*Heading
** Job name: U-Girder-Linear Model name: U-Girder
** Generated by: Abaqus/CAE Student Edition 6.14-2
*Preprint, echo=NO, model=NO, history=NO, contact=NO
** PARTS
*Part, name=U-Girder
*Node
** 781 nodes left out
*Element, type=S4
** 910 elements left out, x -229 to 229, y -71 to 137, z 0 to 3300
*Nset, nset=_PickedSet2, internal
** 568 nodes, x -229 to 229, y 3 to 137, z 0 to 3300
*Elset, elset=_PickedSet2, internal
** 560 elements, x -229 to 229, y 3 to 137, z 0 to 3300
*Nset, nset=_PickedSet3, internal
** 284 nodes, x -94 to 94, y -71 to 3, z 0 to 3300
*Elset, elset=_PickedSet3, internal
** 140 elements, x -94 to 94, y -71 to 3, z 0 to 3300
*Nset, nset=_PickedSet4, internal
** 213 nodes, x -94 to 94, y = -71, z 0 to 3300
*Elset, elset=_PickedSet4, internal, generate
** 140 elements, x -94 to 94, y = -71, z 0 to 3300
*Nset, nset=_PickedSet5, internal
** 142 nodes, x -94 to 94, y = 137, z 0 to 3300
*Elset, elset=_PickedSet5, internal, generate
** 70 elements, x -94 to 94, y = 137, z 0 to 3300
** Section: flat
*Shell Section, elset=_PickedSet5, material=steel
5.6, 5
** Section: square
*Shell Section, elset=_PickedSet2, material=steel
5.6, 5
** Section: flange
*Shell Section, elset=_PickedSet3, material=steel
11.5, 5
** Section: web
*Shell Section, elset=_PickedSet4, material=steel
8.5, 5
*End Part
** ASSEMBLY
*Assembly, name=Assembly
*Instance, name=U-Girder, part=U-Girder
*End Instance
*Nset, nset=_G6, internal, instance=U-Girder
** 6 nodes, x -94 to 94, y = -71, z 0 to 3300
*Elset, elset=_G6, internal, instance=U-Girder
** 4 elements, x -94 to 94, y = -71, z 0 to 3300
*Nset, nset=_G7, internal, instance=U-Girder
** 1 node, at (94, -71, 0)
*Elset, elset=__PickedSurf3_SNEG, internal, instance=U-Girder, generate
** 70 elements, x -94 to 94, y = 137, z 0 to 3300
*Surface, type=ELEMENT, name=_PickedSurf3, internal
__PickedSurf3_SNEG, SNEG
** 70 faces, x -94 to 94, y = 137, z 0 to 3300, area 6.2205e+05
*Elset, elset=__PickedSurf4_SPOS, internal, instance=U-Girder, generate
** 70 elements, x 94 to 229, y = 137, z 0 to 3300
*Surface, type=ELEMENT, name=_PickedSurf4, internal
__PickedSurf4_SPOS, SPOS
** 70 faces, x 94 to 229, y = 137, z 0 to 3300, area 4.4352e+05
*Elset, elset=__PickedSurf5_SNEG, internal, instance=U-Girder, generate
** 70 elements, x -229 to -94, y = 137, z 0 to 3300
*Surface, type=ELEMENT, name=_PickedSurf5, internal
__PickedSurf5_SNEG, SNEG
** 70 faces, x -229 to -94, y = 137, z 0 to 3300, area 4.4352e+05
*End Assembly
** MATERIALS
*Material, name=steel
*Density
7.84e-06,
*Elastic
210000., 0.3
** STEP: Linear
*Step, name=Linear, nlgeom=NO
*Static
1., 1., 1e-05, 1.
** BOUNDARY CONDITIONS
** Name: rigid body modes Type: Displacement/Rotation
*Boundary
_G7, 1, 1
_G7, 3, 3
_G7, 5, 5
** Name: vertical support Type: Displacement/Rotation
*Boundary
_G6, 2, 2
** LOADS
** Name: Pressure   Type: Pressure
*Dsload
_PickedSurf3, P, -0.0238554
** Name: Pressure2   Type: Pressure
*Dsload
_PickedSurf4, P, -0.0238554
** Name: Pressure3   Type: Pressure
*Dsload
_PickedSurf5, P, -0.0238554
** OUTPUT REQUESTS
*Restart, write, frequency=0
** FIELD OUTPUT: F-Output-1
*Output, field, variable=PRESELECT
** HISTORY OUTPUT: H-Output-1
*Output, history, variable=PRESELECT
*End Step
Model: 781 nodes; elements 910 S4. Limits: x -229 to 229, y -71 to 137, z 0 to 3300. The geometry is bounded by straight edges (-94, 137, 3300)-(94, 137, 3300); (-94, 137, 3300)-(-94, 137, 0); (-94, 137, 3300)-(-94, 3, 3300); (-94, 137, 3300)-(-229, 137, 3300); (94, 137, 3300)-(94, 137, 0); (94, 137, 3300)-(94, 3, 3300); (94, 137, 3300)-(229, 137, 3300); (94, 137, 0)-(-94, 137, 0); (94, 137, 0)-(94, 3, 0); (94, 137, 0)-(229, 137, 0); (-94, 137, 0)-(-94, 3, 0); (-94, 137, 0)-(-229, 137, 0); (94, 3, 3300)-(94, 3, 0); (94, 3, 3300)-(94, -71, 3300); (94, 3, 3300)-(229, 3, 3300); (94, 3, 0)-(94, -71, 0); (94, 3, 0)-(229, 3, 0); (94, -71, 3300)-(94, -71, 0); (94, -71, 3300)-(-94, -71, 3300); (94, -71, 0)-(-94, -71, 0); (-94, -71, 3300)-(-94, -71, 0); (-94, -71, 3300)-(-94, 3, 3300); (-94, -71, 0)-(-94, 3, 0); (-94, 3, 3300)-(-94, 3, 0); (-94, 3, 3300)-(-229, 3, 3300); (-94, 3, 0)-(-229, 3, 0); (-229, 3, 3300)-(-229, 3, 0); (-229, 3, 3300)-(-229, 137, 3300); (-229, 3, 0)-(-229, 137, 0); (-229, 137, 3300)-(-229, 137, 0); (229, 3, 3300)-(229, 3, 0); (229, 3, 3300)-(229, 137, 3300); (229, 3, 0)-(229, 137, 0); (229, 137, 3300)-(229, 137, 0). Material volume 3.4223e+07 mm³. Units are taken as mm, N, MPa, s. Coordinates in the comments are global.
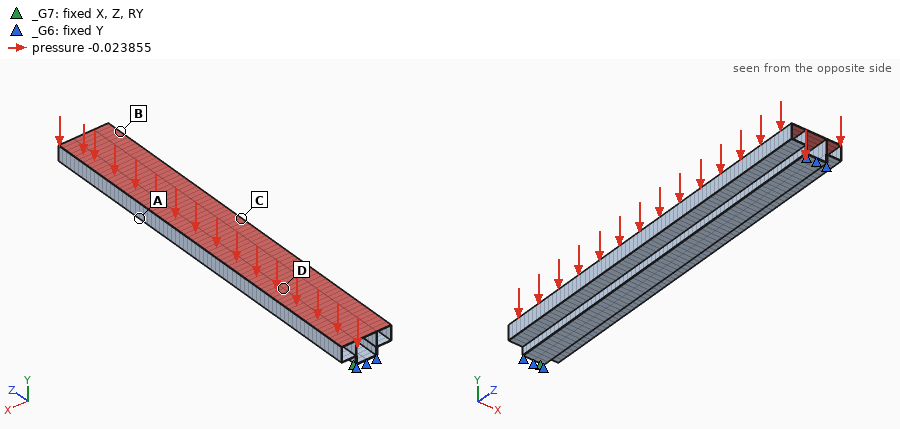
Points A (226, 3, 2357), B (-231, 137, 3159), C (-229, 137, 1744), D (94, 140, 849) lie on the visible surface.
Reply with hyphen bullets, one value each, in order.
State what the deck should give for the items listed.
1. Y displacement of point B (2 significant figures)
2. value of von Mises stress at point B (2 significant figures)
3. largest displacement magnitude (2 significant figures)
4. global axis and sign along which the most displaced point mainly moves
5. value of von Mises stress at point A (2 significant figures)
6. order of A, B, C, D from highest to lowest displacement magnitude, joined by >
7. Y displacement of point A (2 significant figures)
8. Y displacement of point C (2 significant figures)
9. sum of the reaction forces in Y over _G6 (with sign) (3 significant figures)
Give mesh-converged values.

- -0.32 mm
- 6.1 MPa
- 1.5 mm
- -Y
- 8.6 MPa
- C > A > D > B
- -1.1 mm
- -1.4 mm
- 36000 N
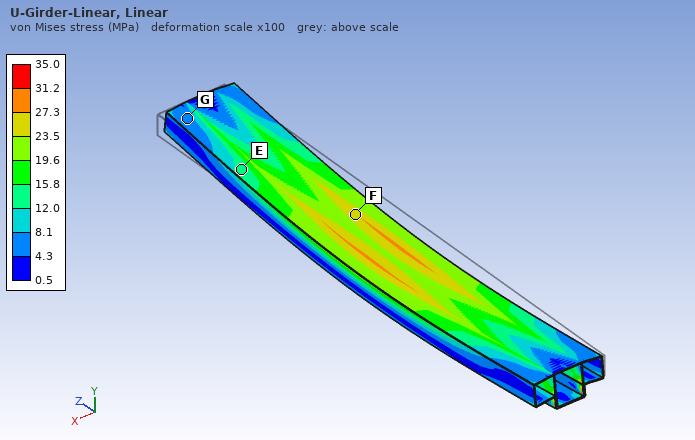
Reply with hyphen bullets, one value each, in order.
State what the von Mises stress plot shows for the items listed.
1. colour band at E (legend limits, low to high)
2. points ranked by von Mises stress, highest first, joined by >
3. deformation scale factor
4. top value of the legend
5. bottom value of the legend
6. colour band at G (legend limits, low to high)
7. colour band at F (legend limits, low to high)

- 12.0 to 15.8 MPa
- F > E > G
- 100
- 35.0 MPa
- 0.5 MPa
- 4.3 to 8.1 MPa
- 23.5 to 27.3 MPa
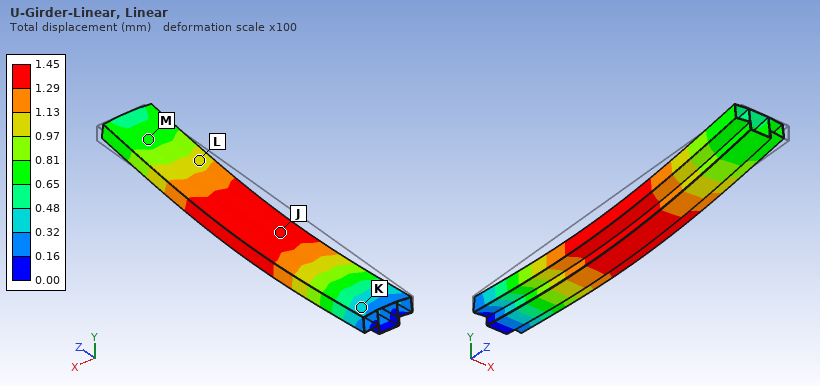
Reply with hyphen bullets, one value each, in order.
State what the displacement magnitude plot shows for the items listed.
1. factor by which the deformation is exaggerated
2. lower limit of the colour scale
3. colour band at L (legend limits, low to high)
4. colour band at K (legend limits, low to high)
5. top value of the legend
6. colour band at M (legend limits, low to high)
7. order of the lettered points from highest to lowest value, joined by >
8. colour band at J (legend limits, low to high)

- 100
- 0.00 mm
- 0.97 to 1.13 mm
- 0.32 to 0.48 mm
- 1.45 mm
- 0.65 to 0.81 mm
- J > L > M > K
- 1.29 to 1.45 mm
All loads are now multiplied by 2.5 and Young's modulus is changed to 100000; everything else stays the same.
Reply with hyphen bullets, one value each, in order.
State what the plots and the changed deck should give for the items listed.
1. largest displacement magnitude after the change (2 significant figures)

- 7.6 mm
